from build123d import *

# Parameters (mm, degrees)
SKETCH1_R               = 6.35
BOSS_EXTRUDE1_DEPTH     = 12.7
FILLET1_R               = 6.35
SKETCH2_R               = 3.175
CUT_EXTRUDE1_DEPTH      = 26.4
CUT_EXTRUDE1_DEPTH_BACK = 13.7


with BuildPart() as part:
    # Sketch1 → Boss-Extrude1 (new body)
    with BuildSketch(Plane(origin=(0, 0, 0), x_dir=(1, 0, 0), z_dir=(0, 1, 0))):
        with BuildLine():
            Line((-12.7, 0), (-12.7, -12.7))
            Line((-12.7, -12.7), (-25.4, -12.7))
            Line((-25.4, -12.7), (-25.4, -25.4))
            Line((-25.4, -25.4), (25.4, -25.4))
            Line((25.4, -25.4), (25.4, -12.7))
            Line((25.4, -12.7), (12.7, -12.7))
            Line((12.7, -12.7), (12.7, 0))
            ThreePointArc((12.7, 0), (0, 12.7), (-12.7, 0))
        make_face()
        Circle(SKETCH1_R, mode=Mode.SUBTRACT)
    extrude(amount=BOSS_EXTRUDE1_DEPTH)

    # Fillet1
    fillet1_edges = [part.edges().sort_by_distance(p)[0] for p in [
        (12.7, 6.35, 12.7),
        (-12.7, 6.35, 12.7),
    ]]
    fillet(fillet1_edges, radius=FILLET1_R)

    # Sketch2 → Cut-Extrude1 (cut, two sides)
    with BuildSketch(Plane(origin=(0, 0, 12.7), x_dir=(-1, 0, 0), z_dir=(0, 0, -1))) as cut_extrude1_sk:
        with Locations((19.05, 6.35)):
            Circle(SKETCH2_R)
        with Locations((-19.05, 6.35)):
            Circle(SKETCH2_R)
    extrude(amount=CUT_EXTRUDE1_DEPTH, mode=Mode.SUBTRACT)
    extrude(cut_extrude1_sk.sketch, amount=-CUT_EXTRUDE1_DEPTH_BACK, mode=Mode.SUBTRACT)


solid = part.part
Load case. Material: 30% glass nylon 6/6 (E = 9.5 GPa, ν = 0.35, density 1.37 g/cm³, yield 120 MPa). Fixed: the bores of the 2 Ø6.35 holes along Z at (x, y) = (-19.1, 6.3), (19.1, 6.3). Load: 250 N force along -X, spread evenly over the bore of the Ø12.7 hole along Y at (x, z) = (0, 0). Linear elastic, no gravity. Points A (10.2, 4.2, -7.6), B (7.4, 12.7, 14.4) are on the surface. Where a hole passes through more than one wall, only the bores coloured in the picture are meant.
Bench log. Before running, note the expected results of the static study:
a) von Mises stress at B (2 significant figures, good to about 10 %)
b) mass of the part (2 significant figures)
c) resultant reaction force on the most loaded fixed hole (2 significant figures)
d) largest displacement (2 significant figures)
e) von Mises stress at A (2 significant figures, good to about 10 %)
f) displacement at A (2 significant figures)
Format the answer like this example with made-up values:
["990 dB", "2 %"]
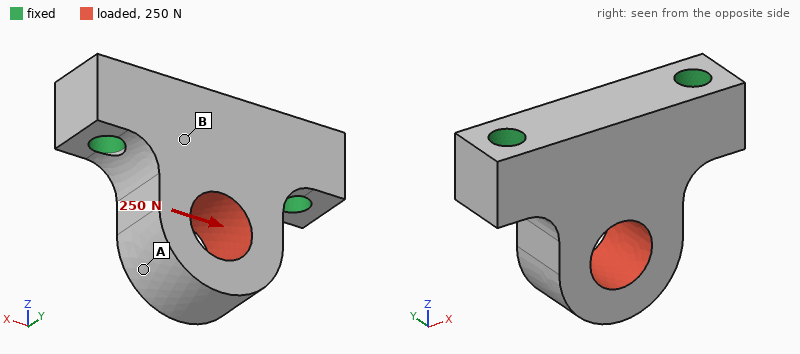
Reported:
["0.61 MPa", "18 g", "180 N", "14 µm", "1.4 MPa", "13 µm"]
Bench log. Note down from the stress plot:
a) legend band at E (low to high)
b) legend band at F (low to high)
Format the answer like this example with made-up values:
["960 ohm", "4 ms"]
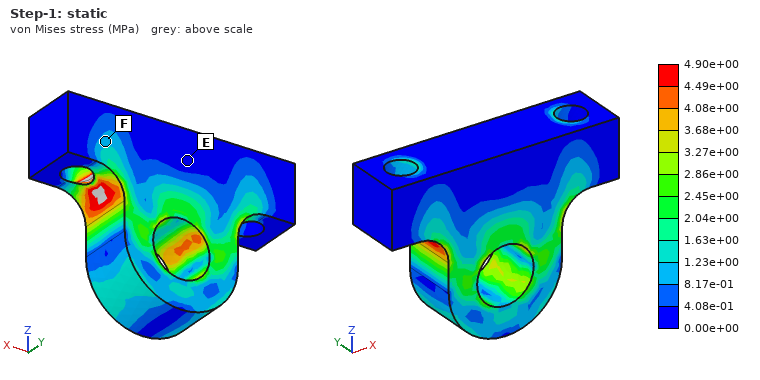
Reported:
["0.00e+00 to 4.08e-01 MPa", "8.17e-01 to 1.23e+00 MPa"]
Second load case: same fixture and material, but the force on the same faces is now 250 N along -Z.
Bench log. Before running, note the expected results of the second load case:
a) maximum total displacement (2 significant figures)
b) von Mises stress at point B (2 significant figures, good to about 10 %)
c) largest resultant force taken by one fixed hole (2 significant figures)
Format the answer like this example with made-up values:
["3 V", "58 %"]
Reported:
["4.6 µm", "0.53 MPa", "140 N"]
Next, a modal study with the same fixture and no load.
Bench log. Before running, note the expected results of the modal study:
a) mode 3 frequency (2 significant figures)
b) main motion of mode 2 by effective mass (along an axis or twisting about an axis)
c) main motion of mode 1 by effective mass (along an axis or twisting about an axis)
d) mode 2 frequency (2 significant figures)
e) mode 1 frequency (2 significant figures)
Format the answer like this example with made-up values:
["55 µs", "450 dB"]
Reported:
["12 kHz", "along X", "along Y", "9100 Hz", "4600 Hz"]
